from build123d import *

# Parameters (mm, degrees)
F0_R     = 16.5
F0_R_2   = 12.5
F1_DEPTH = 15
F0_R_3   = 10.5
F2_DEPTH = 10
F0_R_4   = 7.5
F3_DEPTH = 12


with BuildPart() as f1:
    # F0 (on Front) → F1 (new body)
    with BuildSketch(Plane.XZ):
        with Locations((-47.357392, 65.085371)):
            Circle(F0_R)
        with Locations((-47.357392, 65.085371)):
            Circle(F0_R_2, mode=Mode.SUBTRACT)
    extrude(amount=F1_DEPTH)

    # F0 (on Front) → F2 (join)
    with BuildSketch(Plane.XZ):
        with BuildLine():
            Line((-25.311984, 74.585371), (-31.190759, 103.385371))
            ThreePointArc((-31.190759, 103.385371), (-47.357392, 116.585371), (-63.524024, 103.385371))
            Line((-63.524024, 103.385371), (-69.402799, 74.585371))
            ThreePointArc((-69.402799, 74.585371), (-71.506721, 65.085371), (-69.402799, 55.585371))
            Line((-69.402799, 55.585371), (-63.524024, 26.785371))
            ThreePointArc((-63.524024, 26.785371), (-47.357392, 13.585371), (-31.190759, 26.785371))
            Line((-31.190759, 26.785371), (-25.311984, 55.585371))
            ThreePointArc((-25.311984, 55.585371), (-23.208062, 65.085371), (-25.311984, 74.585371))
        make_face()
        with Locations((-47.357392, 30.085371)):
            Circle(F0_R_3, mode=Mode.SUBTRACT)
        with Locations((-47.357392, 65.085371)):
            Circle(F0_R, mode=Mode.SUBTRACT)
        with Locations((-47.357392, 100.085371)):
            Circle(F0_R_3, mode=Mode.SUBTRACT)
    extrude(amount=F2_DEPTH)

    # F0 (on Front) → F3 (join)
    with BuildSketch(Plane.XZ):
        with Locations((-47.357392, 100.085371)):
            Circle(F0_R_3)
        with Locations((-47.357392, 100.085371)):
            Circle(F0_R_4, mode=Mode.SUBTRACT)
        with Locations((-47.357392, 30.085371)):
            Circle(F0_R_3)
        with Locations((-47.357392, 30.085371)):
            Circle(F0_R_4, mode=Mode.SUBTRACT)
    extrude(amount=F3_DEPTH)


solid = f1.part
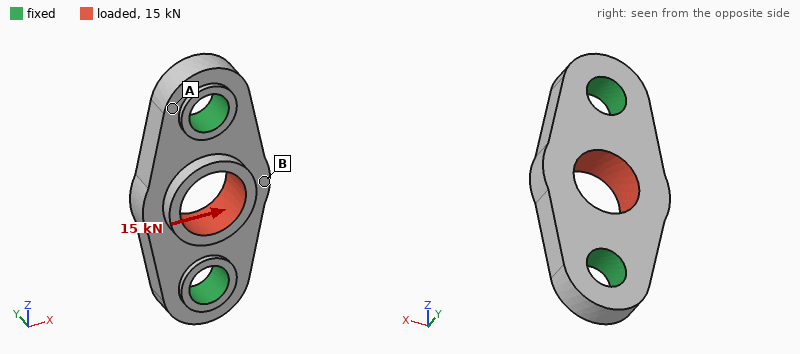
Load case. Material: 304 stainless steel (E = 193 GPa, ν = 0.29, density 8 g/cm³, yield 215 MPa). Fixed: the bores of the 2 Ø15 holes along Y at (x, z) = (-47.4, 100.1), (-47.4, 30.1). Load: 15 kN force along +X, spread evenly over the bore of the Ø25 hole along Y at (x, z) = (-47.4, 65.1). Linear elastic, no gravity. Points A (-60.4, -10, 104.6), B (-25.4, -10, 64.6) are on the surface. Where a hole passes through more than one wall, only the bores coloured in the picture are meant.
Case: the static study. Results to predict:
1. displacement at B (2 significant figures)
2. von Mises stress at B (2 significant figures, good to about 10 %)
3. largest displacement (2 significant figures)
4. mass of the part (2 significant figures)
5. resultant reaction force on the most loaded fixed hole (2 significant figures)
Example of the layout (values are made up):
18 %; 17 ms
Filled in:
13 µm; 26 MPa; 15 µm; 250 g; 7.5 kN
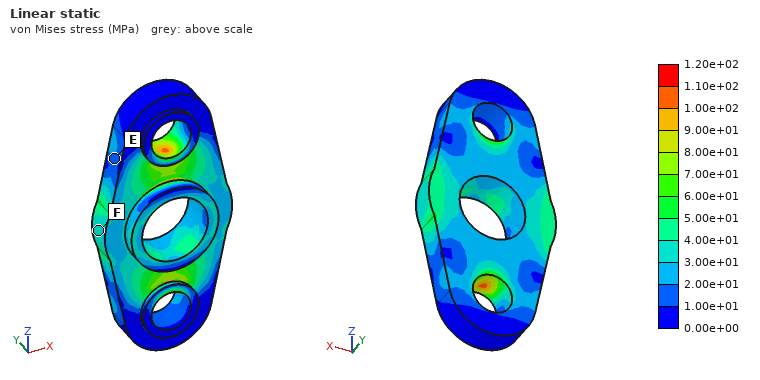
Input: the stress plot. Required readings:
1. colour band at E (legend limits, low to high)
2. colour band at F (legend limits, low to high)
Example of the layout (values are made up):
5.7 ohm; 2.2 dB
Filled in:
1.00e+01 to 2.00e+01 MPa; 3.00e+01 to 4.00e+01 MPa
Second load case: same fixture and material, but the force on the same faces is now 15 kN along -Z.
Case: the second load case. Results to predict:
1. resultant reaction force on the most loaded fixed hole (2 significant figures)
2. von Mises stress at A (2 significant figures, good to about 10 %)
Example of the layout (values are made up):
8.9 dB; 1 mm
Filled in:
7.5 kN; 7.1 MPa
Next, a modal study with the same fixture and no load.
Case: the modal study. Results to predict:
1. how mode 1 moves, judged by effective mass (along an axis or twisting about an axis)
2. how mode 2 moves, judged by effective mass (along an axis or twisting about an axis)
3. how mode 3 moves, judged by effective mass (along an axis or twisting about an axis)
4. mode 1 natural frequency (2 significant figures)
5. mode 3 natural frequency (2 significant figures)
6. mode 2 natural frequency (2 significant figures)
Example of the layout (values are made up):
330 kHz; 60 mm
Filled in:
twisting about Z; along Y; along X; 11 kHz; 21 kHz; 11 kHz
